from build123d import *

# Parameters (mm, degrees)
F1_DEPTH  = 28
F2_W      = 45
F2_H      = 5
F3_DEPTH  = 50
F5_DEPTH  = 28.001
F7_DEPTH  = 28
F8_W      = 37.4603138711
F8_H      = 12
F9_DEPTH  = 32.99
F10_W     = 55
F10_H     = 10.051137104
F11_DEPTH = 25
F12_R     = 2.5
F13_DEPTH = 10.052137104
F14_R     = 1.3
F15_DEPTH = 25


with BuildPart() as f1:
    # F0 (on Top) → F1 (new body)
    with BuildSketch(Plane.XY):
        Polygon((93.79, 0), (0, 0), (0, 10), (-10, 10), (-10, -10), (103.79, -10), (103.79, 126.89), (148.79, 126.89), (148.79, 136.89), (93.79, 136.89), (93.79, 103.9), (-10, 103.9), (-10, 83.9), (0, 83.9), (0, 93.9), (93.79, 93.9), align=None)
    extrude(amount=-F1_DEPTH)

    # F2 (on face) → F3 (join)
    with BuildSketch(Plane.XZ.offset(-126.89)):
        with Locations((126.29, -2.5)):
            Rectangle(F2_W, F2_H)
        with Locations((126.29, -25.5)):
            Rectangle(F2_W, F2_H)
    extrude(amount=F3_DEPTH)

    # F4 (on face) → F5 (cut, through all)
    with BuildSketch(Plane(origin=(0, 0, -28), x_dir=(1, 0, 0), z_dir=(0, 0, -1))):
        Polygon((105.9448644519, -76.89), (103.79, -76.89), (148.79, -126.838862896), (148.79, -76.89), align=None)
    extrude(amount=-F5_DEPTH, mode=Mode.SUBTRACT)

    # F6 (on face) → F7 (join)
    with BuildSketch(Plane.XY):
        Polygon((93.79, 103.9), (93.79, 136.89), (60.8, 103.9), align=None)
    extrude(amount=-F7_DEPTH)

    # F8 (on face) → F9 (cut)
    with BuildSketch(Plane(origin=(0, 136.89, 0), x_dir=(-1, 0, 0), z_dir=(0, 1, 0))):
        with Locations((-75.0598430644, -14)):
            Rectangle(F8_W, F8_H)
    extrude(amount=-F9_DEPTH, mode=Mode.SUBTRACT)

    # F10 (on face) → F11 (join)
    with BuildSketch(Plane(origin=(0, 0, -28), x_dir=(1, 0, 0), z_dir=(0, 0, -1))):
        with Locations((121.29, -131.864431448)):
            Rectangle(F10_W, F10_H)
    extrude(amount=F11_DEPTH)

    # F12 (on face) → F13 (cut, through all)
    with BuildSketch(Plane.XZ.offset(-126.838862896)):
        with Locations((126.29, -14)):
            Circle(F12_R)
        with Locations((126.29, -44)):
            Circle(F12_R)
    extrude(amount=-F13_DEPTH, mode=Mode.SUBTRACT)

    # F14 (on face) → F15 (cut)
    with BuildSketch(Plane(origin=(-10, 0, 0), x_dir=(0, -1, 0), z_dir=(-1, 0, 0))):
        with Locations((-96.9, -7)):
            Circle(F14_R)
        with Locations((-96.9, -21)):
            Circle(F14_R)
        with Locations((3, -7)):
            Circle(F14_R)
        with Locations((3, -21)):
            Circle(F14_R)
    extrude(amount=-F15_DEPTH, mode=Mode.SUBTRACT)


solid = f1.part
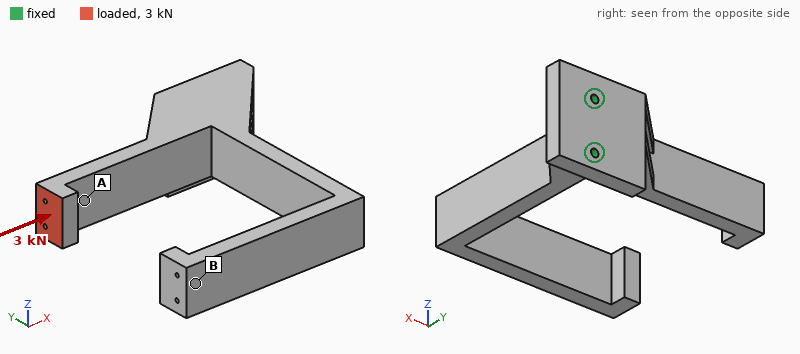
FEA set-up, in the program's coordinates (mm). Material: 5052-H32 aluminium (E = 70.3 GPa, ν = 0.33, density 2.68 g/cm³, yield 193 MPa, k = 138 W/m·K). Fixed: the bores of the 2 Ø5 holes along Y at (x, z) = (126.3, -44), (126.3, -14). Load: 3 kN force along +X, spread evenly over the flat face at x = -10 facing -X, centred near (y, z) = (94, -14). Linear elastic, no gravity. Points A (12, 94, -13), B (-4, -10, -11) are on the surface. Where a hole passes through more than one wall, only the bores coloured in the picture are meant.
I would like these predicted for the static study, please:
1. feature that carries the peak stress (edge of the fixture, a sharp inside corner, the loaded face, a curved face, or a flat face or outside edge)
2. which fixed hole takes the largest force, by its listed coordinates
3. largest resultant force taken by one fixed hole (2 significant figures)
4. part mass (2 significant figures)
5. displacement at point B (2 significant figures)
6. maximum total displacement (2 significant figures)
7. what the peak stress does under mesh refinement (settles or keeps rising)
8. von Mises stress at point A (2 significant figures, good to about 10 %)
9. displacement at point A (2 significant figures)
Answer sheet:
edge of the fixture
(126.3, -14)
2.9 kN
400 g
0.60 mm
0.82 mm
keeps rising
44 MPa
0.57 mm
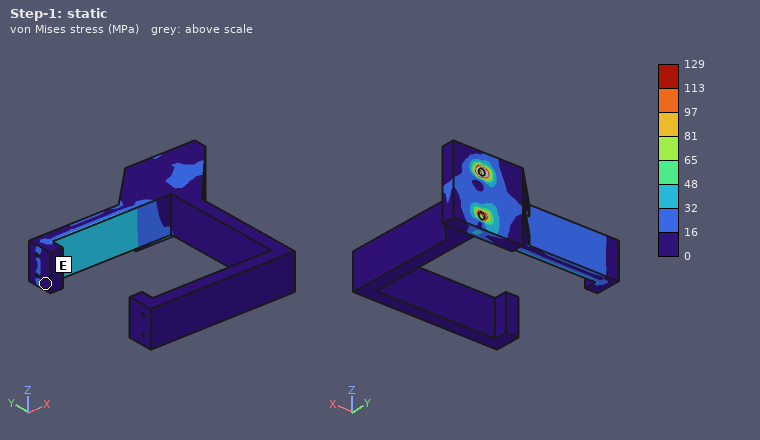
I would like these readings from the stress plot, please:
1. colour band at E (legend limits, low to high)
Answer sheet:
0 to 16 MPa
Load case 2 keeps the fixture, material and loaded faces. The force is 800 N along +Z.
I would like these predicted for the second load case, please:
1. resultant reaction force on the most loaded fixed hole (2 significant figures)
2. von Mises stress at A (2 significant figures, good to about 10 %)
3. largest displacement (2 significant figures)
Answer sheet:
3.5 kN
17 MPa
0.39 mm
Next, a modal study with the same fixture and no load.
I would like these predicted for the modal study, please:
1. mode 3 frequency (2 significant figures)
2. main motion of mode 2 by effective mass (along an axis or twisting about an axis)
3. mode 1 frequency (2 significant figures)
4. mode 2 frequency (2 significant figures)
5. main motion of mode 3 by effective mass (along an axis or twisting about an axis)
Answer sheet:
590 Hz
along Z
230 Hz
340 Hz
along X
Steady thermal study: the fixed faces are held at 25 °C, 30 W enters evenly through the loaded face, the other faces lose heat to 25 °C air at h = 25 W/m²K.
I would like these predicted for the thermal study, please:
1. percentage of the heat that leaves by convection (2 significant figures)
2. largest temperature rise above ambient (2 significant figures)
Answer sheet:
41 %
68 K
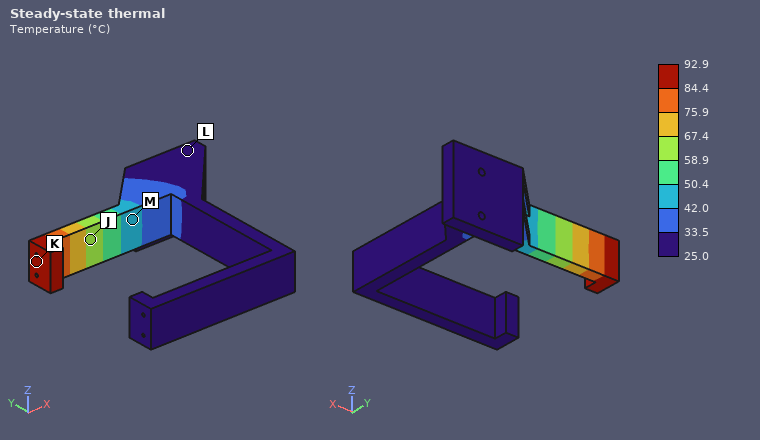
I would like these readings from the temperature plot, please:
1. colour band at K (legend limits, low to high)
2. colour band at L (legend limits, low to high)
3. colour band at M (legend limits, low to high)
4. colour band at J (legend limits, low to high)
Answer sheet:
84.4 to 92.9 °C
25.0 to 33.5 °C
42.0 to 50.4 °C
58.9 to 67.4 °C
